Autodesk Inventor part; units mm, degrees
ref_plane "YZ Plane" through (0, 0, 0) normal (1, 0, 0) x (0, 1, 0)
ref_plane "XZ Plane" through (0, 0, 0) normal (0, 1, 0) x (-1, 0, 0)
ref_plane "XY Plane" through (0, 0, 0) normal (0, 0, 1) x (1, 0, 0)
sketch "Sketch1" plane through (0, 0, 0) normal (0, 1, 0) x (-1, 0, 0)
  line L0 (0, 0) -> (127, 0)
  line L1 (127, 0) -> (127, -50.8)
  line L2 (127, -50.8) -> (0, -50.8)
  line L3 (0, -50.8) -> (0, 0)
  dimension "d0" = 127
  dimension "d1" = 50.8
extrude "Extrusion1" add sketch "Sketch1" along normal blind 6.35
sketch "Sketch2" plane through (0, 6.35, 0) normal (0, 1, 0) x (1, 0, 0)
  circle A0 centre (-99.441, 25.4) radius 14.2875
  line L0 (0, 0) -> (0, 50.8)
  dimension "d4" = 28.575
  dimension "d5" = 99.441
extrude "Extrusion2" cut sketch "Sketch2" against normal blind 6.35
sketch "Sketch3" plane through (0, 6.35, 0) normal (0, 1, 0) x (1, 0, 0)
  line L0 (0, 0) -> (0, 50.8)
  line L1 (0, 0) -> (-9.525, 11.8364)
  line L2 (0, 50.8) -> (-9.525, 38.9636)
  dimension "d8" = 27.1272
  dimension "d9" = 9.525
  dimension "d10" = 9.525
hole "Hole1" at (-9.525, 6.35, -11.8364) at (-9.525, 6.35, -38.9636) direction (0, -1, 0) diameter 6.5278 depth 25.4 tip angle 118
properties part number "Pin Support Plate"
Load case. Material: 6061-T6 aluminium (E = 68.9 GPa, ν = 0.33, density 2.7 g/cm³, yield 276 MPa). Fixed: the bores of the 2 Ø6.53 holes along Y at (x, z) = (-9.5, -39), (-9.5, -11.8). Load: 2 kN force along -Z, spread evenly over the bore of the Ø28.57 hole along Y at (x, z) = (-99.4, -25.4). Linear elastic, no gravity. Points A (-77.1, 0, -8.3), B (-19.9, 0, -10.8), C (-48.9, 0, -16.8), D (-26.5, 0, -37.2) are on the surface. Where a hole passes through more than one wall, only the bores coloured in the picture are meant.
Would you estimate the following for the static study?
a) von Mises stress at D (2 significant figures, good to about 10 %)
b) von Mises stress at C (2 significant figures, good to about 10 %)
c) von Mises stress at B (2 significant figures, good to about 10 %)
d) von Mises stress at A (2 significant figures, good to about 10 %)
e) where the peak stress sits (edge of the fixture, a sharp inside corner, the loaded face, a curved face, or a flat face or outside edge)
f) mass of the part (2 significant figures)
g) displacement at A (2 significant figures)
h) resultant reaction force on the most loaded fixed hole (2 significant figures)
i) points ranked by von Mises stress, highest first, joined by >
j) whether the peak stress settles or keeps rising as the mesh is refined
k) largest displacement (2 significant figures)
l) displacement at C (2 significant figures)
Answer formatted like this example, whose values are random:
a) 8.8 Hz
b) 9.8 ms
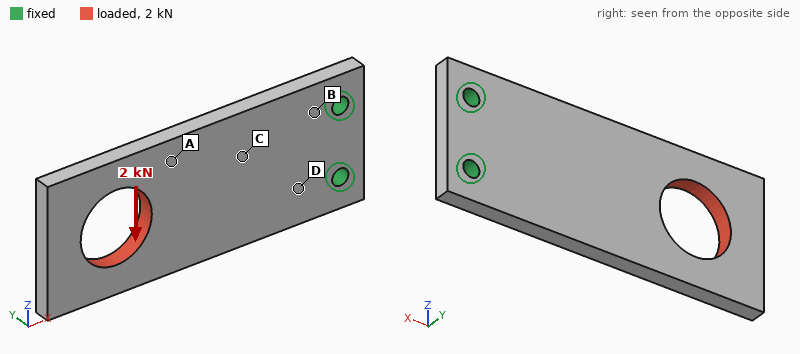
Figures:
a) 34 MPa
b) 19 MPa
c) 49 MPa
d) 9.4 MPa
e) edge of the fixture
f) 98 g
g) 0.10 mm
h) 5.8 kN
i) B > D > C > A
j) keeps rising
k) 0.23 mm
l) 0.046 mm
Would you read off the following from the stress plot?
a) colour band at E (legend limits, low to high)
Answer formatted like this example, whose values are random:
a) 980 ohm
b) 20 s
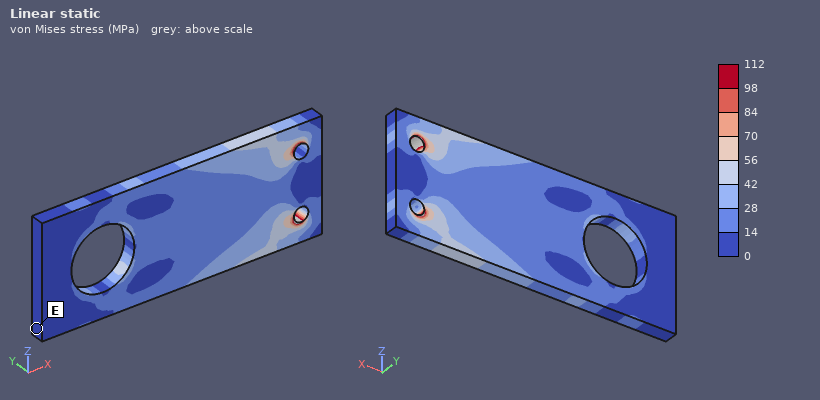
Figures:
a) 0 to 14 MPa
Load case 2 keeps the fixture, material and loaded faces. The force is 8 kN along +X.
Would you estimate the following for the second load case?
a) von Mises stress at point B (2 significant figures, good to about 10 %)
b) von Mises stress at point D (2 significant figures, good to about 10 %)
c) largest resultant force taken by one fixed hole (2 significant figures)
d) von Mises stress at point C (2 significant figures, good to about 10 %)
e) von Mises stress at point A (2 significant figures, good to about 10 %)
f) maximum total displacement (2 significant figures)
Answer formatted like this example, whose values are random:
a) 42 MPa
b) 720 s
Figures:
a) 34 MPa
b) 28 MPa
c) 4.0 kN
d) 24 MPa
e) 31 MPa
f) 58 µm
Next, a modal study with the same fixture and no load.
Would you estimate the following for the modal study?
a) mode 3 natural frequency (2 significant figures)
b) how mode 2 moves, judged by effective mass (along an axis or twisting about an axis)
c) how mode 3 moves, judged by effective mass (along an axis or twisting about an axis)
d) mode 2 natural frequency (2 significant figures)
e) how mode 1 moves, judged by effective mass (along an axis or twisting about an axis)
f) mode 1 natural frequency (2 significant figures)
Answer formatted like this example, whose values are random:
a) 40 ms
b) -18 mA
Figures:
a) 2200 Hz
b) twisting about X
c) along Y
d) 1700 Hz
e) along Y
f) 430 Hz
